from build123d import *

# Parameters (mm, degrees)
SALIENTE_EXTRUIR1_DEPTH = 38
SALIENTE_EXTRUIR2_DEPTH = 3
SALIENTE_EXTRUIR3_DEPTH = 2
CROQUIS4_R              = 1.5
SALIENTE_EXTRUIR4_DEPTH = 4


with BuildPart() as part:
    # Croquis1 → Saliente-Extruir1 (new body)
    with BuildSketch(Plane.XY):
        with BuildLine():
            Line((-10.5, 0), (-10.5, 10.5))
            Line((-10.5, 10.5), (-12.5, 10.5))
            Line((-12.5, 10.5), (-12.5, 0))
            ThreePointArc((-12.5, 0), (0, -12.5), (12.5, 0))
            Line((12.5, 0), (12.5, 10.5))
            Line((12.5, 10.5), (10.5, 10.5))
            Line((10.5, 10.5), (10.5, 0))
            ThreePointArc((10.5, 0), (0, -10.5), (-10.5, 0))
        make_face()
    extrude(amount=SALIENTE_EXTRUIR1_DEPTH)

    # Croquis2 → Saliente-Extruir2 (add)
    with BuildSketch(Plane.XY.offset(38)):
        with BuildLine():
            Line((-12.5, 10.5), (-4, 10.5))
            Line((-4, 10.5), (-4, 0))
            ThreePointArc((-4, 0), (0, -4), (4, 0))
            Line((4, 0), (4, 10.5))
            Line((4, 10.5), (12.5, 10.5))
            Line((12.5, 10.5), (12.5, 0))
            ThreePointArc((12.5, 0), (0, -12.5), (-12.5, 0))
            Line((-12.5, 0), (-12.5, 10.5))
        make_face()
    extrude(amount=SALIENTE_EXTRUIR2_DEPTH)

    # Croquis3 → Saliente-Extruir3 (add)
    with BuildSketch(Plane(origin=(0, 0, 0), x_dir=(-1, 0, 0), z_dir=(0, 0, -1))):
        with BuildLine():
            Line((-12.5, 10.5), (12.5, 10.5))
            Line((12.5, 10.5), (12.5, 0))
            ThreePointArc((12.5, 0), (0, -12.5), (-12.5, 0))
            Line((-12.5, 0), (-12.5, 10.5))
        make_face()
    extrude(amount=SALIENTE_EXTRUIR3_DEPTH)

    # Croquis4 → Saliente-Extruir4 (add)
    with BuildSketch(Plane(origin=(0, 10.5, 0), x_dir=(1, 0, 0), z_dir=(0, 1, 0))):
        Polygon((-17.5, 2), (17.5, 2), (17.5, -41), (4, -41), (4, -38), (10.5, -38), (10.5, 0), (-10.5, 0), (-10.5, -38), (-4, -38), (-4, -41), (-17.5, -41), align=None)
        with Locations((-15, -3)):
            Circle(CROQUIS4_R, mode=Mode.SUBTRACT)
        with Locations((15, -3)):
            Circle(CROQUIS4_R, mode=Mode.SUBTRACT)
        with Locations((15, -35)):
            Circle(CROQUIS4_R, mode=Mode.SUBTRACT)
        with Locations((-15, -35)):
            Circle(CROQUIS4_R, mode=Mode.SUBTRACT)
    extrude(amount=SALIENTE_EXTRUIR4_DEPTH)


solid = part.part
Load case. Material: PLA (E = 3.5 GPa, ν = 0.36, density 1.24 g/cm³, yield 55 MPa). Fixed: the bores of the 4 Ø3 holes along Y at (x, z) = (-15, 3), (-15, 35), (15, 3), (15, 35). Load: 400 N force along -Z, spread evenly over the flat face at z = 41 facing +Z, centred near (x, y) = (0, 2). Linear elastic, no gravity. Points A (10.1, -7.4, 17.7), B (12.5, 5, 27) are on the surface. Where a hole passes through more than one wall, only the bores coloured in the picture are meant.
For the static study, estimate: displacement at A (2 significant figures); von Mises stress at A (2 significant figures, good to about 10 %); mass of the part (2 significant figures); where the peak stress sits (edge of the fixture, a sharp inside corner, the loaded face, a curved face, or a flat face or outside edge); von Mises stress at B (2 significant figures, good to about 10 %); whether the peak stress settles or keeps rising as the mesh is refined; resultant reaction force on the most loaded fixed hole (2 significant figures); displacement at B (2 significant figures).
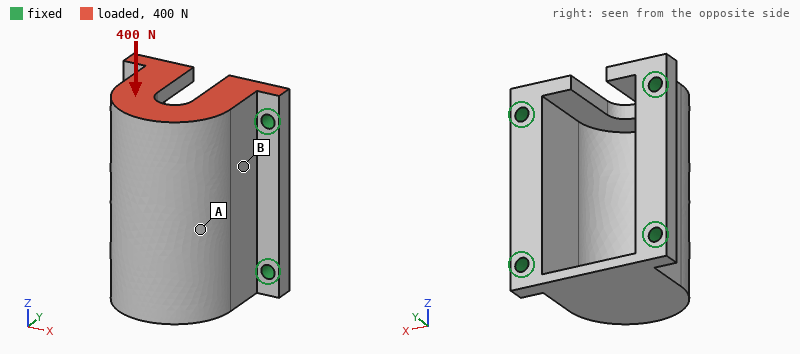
0.038 mm
1.7 MPa
11 g
edge of the fixture
4.3 MPa
keeps rising
140 N
0.028 mm
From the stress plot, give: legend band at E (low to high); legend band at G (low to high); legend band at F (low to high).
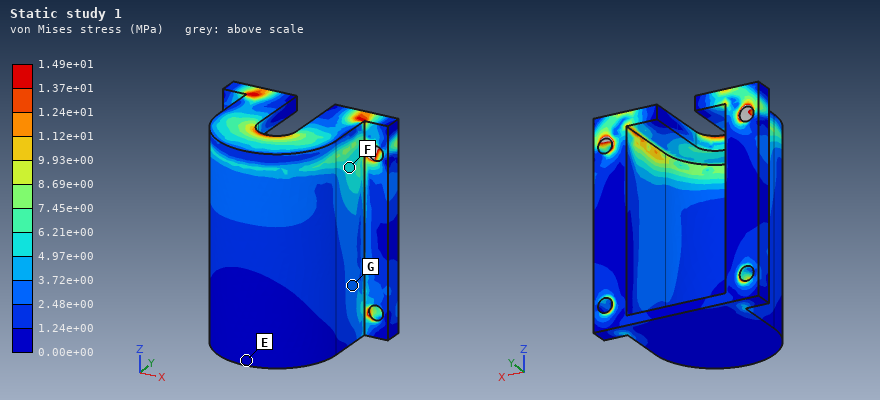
0.00e+00 to 1.24e+00 MPa
2.48e+00 to 3.72e+00 MPa
4.97e+00 to 6.21e+00 MPa
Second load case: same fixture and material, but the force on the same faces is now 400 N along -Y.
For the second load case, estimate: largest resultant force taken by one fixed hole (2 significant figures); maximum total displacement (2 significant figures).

230 N
85 µm
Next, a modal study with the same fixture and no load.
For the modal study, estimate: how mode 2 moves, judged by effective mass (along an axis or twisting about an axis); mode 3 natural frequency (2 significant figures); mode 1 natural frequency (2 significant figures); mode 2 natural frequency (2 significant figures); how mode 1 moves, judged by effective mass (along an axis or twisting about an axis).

along Z
5100 Hz
3200 Hz
4600 Hz
along X
